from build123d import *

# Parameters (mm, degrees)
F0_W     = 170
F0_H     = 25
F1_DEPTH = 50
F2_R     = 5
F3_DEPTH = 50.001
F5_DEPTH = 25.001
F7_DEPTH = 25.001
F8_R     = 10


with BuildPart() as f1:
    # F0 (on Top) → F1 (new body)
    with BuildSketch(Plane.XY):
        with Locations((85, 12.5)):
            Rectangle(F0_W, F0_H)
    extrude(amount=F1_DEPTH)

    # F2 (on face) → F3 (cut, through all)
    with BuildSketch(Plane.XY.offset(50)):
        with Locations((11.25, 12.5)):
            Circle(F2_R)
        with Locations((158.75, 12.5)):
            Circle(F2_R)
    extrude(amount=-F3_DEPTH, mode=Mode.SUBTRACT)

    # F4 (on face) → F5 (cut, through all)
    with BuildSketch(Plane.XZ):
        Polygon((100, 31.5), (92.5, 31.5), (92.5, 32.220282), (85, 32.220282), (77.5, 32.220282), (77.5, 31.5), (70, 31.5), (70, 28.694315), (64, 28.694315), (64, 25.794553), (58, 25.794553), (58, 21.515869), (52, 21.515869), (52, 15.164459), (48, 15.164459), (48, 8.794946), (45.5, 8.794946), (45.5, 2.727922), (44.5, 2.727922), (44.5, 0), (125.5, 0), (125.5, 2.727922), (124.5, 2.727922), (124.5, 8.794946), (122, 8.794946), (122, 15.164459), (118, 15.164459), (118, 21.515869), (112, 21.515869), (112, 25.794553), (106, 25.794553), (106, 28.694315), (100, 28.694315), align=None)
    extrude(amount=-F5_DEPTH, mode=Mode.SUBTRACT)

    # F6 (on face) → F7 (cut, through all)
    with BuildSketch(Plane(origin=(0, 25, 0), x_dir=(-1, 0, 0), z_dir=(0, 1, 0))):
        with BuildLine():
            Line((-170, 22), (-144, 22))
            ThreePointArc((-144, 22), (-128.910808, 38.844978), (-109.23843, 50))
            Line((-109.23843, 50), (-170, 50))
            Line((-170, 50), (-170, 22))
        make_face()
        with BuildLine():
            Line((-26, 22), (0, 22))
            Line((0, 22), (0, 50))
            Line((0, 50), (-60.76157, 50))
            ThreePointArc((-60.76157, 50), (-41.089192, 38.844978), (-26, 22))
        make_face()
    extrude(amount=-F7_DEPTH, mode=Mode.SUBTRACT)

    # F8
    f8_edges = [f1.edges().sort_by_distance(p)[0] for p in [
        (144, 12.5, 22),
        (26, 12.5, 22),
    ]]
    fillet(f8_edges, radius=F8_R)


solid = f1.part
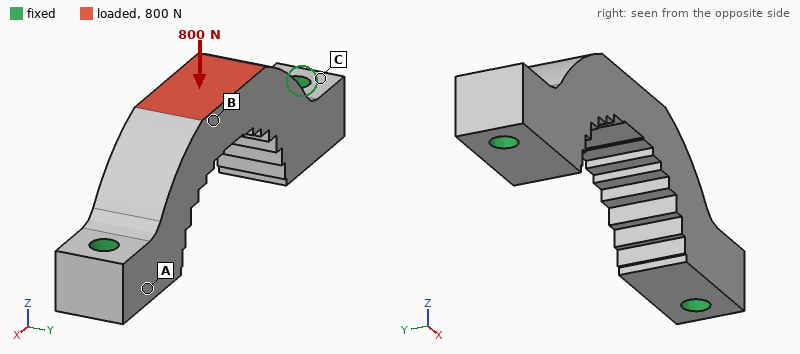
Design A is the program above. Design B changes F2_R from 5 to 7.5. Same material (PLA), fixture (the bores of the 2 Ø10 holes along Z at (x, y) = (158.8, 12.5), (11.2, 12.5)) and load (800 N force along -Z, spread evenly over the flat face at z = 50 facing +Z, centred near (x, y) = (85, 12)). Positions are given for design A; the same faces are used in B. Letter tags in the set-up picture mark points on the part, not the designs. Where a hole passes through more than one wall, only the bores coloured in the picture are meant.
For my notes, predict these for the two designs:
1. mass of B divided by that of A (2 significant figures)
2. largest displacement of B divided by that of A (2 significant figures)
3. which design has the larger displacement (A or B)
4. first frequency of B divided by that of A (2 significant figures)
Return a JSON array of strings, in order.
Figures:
["0.96", "0.91", "A", "1.1"]
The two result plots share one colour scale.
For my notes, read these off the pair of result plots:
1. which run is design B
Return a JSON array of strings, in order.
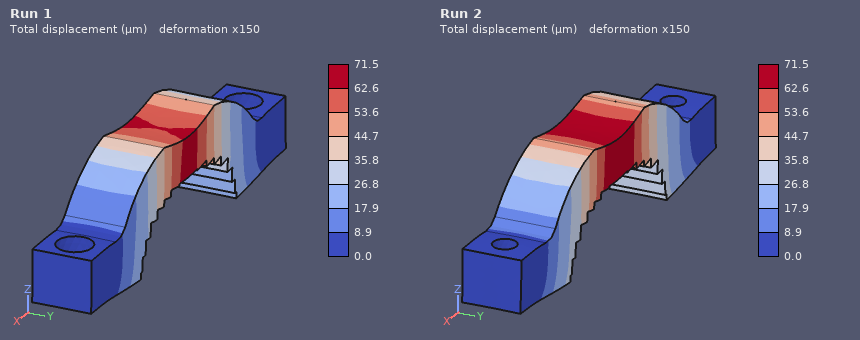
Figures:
["Run 1"]
